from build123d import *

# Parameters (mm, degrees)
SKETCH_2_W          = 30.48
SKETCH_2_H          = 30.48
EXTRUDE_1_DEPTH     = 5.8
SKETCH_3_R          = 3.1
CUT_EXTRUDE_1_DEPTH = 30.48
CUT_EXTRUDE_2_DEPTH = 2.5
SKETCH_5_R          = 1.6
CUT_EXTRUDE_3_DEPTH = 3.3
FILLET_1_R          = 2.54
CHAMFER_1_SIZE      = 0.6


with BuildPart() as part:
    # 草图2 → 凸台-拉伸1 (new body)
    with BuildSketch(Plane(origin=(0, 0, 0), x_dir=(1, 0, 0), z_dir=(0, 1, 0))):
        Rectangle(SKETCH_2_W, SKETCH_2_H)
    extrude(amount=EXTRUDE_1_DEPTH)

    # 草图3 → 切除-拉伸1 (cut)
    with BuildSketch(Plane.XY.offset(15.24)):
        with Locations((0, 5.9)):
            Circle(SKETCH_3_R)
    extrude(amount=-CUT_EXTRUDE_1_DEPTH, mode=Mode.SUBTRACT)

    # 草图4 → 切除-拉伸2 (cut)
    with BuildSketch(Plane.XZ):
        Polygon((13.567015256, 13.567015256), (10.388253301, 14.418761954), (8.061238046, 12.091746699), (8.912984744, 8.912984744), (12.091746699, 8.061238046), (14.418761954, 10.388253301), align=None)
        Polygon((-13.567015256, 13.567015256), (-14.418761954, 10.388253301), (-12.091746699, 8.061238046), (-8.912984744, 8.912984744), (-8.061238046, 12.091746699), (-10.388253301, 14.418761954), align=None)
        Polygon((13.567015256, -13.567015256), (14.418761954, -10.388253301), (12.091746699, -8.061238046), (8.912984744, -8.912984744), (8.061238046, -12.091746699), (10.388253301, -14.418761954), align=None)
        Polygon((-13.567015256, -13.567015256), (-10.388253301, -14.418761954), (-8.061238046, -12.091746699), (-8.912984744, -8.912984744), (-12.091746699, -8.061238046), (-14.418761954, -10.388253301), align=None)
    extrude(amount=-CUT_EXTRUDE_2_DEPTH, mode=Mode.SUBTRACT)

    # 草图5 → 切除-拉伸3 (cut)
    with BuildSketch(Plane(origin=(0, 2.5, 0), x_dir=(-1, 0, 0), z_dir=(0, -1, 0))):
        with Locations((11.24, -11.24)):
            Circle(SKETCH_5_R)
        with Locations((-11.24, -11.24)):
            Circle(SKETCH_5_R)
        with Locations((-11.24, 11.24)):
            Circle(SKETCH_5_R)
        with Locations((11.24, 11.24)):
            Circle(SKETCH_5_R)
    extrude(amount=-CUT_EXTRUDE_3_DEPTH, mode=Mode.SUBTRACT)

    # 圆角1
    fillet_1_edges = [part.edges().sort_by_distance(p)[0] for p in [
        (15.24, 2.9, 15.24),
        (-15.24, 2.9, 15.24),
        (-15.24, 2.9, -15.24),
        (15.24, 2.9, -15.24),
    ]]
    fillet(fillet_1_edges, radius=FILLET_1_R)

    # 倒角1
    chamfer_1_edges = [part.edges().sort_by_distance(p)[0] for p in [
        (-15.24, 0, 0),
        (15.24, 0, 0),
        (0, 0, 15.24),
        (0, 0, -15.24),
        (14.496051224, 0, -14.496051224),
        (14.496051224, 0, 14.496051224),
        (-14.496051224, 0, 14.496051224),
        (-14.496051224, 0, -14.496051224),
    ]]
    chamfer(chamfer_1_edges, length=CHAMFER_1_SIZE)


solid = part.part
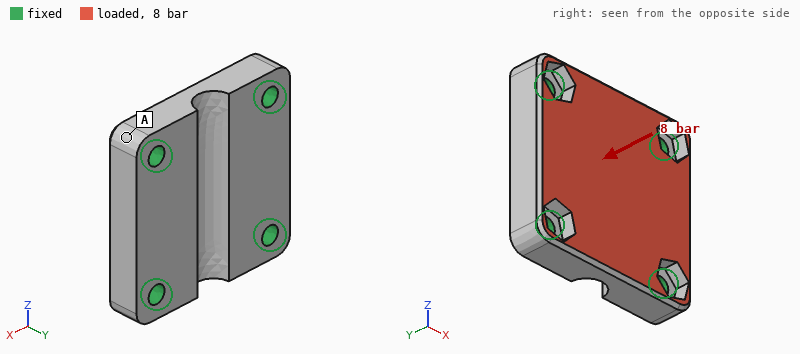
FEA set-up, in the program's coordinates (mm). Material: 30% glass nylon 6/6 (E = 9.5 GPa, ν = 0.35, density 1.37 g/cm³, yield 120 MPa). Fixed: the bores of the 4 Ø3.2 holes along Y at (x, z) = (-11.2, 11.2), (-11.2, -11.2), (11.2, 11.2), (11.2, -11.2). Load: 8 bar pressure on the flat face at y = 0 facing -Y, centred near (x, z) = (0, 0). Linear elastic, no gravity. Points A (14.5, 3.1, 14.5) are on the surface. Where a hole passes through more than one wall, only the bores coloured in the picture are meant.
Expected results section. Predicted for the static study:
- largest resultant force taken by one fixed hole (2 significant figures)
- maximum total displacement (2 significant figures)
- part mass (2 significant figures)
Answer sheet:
190 N
21 µm
6.2 g
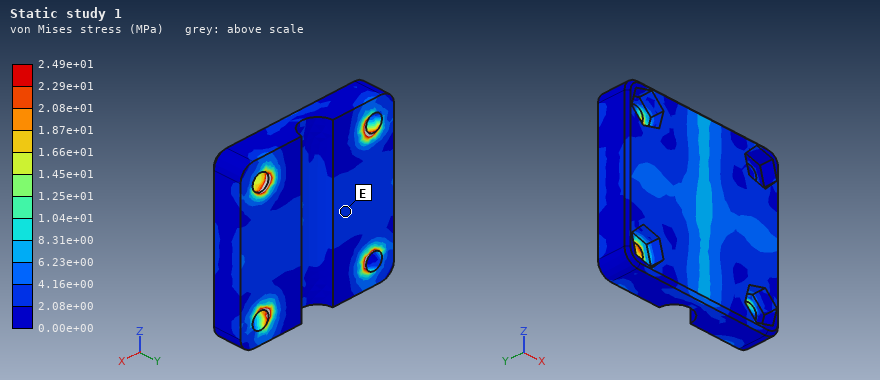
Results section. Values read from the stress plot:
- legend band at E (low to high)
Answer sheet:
2.08e+00 to 4.16e+00 MPa
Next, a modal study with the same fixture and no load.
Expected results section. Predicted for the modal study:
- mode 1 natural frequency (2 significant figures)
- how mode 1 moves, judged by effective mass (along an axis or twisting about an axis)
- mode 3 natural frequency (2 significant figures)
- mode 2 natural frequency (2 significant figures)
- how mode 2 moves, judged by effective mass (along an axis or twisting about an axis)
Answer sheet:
15 kHz
along Y
22 kHz
21 kHz
twisting about Z
